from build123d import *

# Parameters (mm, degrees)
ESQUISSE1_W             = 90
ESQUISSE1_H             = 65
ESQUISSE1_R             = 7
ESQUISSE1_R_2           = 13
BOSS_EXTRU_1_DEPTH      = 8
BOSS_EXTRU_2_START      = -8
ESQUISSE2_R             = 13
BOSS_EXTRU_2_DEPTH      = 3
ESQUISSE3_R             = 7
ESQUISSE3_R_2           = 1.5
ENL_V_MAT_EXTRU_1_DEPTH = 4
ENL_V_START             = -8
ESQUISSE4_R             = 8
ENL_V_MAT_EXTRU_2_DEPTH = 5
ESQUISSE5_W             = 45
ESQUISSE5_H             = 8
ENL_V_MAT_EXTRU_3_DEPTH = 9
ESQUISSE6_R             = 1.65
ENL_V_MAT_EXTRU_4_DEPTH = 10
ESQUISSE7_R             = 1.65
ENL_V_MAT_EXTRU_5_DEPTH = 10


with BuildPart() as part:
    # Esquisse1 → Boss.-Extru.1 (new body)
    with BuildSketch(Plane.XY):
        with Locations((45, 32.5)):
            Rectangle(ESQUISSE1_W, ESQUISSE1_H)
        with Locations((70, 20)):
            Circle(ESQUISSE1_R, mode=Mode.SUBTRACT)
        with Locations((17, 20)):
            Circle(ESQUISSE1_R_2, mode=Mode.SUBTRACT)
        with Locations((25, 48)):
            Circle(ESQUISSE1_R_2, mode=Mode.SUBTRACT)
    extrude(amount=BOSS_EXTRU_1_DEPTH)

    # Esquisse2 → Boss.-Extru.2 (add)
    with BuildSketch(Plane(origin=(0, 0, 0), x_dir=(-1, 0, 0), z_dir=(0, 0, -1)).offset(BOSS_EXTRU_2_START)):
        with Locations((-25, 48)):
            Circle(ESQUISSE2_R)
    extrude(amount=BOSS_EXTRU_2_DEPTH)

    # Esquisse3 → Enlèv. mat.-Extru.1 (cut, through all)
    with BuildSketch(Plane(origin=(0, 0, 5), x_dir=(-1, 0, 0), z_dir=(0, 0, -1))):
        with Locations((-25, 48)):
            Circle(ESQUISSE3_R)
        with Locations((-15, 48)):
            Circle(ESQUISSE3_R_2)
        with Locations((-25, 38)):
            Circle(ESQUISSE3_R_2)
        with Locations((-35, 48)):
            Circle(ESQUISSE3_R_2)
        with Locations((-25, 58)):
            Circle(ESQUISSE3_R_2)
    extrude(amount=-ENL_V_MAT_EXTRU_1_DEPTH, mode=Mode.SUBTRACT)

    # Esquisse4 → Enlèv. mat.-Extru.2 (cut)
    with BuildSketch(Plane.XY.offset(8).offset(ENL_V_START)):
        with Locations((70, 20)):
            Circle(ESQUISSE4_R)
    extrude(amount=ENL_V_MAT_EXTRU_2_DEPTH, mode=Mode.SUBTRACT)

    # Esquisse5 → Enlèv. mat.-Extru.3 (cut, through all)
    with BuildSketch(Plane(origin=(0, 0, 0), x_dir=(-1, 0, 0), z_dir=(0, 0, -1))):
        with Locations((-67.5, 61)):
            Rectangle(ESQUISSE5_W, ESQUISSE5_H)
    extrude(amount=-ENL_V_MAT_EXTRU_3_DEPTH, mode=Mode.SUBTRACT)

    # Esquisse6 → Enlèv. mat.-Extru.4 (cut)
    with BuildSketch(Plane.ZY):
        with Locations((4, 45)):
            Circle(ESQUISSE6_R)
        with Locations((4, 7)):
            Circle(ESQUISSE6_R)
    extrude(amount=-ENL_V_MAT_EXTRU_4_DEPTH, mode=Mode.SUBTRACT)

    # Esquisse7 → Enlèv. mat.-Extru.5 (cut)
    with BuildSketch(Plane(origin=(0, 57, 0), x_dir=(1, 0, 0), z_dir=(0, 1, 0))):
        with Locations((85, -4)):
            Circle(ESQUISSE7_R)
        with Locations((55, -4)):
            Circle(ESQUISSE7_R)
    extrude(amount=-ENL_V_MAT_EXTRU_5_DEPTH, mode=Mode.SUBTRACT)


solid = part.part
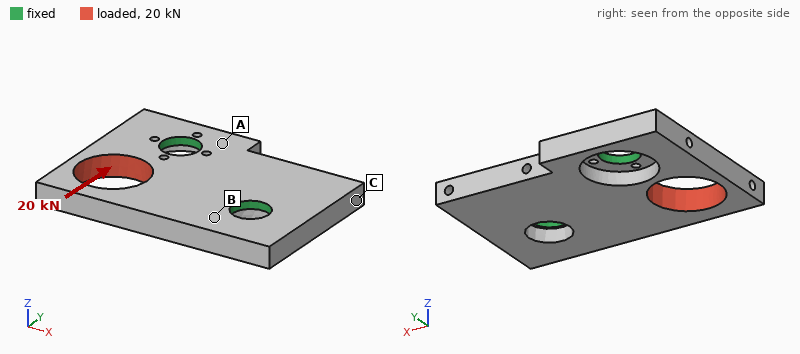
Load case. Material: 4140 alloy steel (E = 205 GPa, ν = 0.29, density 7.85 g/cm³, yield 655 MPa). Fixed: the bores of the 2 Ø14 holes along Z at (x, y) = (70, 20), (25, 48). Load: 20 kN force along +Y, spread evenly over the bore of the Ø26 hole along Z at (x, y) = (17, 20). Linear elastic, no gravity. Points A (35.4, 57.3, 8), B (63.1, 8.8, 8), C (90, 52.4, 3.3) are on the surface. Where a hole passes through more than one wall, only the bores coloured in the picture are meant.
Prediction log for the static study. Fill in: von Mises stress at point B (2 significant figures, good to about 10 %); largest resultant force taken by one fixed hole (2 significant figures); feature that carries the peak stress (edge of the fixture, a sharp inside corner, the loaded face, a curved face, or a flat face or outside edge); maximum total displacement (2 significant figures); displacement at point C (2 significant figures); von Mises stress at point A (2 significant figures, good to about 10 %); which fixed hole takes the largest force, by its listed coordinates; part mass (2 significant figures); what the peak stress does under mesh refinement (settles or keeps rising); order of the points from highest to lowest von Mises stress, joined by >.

65 MPa
19 kN
a sharp inside corner
0.10 mm
0.021 mm
130 MPa
(25, 48)
270 g
keeps rising
A > B > C
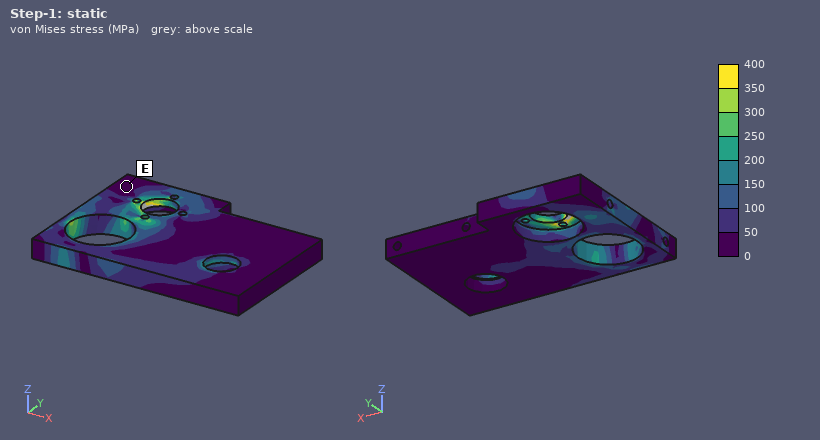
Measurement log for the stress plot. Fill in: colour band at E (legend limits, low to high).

0 to 50 MPa
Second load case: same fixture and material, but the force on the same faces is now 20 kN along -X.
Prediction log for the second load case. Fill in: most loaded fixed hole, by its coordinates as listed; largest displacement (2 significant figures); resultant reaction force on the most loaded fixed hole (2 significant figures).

(70, 20)
74 µm
13 kN
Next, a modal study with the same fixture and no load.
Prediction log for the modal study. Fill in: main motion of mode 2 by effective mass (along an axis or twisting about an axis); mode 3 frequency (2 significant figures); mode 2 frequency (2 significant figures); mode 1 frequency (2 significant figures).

along Z
6400 Hz
5200 Hz
3000 Hz
